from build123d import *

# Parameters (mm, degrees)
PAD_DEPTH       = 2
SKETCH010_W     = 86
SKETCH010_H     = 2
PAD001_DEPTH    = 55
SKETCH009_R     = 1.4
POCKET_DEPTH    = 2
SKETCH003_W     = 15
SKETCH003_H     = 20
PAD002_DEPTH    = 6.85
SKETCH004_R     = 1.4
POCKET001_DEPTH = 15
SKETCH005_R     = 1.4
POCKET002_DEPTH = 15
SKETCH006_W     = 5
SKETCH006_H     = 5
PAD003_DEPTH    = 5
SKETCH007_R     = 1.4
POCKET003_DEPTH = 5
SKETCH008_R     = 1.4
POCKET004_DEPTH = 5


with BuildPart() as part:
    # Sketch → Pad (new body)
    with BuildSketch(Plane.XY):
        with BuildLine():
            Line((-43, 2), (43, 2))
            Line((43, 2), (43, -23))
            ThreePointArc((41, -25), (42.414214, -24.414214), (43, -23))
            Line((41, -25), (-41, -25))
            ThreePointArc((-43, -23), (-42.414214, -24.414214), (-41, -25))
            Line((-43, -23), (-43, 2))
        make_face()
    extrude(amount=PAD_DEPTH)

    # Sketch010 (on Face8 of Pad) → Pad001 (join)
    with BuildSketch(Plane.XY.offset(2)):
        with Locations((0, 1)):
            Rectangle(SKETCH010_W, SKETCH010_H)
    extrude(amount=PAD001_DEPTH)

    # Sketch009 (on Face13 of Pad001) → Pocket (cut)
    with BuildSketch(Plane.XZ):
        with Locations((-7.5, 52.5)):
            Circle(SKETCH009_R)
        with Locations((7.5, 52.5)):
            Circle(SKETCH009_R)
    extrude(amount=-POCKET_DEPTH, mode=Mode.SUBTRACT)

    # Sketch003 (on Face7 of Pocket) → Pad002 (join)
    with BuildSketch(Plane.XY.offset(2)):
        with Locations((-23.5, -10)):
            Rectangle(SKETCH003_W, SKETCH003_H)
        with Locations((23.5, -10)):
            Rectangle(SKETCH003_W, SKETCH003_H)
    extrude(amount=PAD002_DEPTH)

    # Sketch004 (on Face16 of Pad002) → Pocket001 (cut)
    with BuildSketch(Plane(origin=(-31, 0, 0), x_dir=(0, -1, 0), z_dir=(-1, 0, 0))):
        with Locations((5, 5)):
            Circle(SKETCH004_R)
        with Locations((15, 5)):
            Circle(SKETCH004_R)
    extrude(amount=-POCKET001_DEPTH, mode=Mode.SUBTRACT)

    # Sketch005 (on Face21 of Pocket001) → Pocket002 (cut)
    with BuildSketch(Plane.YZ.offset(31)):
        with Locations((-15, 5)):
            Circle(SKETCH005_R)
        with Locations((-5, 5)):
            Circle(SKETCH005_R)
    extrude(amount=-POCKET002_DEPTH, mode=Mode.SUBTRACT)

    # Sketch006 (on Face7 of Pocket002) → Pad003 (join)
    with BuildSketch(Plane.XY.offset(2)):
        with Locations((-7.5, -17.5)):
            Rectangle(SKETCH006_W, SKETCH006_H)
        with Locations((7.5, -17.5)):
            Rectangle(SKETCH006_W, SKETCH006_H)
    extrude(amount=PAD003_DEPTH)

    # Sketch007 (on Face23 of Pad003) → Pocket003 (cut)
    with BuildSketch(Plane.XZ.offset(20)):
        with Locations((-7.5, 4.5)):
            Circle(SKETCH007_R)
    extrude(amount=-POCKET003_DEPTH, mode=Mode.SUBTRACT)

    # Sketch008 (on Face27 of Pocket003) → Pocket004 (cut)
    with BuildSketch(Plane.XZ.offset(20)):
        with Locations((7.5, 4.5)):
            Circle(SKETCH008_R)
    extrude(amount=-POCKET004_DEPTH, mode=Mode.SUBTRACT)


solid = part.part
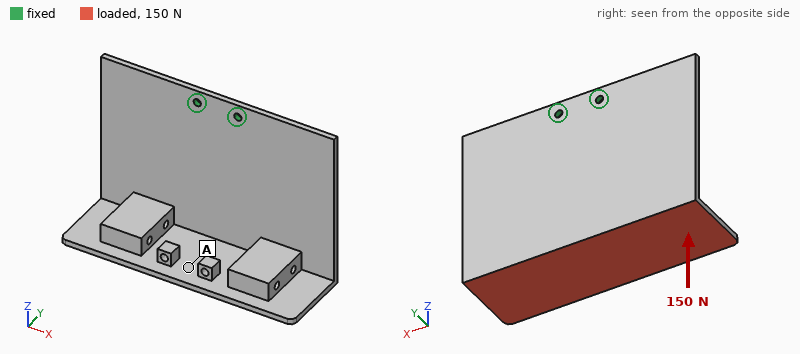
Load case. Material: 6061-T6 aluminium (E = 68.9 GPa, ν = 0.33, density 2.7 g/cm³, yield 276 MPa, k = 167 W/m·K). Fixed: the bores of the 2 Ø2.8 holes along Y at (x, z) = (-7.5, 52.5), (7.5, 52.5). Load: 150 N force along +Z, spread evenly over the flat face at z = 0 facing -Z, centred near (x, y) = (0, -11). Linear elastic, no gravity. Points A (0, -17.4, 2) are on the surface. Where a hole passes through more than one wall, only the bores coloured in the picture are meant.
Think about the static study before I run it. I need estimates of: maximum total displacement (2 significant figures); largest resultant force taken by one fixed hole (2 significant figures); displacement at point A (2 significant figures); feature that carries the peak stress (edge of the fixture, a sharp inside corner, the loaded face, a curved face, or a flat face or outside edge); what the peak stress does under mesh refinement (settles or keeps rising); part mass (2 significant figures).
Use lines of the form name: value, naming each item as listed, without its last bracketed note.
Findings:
maximum total displacement: 1.1 mm
largest resultant force taken by one fixed hole: 76 N
displacement at point A: 0.93 mm
feature that carries the peak stress: edge of the fixture
what the peak stress does under mesh refinement: keeps rising
part mass: 49 g
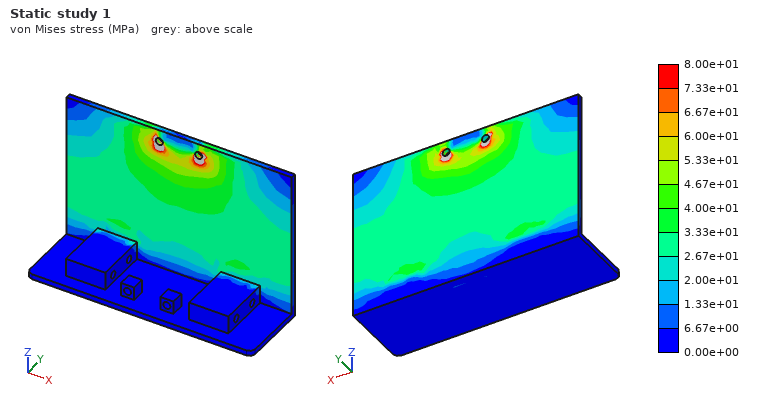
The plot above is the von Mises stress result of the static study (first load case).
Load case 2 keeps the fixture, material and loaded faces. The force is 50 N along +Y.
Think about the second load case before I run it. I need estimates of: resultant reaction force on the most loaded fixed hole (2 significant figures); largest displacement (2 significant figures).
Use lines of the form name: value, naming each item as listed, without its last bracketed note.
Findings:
resultant reaction force on the most loaded fixed hole: 25 N
largest displacement: 1.1 mm
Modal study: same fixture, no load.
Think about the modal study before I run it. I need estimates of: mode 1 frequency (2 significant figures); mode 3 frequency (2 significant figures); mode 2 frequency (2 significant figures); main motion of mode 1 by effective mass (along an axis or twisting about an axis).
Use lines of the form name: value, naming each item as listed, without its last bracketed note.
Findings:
mode 1 frequency: 220 Hz
mode 3 frequency: 1200 Hz
mode 2 frequency: 380 Hz
main motion of mode 1 by effective mass: along Y
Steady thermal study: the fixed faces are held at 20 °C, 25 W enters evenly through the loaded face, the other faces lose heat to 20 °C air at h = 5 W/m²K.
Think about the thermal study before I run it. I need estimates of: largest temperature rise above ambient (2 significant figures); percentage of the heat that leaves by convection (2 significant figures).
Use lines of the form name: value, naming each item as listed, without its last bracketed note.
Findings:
largest temperature rise above ambient: 61 K
percentage of the heat that leaves by convection: 11 %
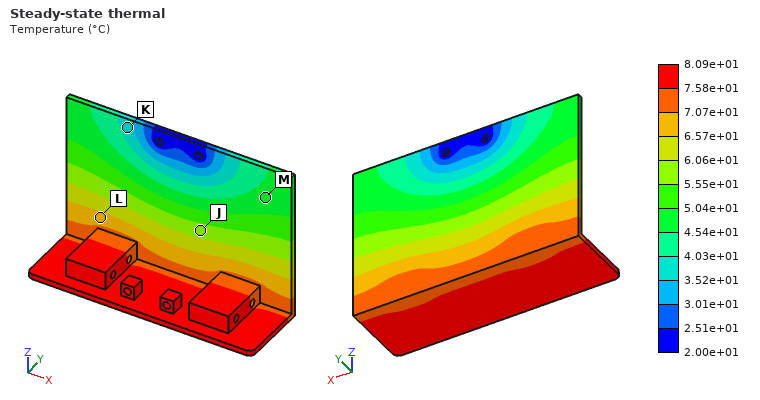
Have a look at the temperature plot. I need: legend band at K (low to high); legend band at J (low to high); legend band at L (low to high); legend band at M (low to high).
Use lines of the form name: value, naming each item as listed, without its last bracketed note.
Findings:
legend band at K: 3.52e+01 to 4.03e+01 °C
legend band at J: 5.55e+01 to 6.06e+01 °C
legend band at L: 6.57e+01 to 7.07e+01 °C
legend band at M: 4.54e+01 to 5.04e+01 °C
